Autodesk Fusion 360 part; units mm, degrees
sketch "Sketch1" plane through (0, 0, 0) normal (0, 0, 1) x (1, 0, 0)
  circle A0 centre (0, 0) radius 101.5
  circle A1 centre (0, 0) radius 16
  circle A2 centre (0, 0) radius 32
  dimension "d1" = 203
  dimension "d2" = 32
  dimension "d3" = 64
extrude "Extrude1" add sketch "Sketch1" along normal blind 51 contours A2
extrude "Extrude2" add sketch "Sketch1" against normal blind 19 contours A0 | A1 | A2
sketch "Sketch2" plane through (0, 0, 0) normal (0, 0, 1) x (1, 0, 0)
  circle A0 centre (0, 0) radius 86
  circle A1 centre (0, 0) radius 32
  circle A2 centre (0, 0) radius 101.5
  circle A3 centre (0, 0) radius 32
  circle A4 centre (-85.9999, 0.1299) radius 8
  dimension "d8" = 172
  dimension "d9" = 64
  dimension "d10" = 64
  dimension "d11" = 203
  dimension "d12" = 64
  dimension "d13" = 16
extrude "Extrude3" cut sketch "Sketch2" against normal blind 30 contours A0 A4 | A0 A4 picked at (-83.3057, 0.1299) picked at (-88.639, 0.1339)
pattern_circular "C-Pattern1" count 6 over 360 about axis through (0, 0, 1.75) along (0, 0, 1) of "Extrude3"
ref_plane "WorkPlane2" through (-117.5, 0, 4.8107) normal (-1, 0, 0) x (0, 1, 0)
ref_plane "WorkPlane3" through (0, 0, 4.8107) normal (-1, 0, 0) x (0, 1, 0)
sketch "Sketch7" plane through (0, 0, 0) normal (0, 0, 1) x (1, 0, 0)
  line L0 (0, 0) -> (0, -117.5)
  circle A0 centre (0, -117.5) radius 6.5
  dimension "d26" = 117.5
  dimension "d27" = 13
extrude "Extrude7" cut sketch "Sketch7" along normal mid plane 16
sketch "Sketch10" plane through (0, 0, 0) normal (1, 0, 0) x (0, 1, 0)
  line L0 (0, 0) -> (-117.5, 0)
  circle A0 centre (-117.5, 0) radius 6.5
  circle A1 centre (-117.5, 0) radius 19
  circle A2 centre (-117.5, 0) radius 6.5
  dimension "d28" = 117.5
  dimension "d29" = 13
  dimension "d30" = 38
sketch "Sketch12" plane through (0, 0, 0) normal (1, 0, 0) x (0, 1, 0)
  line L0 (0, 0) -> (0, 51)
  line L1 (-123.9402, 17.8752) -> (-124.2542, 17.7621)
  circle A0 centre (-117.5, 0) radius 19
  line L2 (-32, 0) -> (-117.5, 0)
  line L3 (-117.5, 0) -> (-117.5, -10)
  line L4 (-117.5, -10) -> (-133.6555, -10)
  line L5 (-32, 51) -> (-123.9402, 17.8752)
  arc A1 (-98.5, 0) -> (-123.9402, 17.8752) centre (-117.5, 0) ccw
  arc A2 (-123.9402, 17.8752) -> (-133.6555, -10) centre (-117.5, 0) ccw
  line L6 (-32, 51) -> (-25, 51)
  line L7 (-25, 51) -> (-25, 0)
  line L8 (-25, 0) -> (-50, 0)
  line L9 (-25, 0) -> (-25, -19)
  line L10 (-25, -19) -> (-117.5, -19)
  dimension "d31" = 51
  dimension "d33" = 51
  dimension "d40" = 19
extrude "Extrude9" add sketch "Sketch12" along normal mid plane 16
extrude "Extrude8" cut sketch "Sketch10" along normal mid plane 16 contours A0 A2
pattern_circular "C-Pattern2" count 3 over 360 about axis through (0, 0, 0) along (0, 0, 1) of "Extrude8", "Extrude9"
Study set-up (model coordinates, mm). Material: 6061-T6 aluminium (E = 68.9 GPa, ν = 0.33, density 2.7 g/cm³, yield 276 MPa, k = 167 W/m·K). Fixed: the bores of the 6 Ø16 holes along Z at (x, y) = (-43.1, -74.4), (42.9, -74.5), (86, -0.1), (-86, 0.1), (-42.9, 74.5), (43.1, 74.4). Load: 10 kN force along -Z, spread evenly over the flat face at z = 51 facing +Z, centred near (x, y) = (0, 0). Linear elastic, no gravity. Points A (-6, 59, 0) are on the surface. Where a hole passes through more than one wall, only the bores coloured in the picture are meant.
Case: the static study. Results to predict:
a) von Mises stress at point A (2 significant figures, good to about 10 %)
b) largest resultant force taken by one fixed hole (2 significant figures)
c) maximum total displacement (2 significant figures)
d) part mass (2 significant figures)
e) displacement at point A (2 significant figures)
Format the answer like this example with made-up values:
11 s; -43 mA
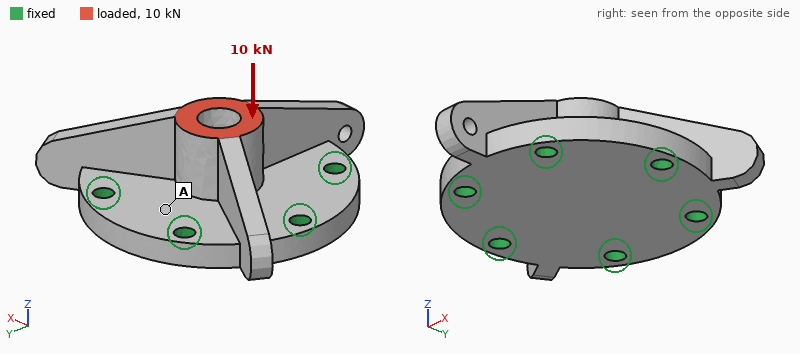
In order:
1.8 MPa; 1.8 kN; 13 µm; 2.4 kg; 4.2 µm
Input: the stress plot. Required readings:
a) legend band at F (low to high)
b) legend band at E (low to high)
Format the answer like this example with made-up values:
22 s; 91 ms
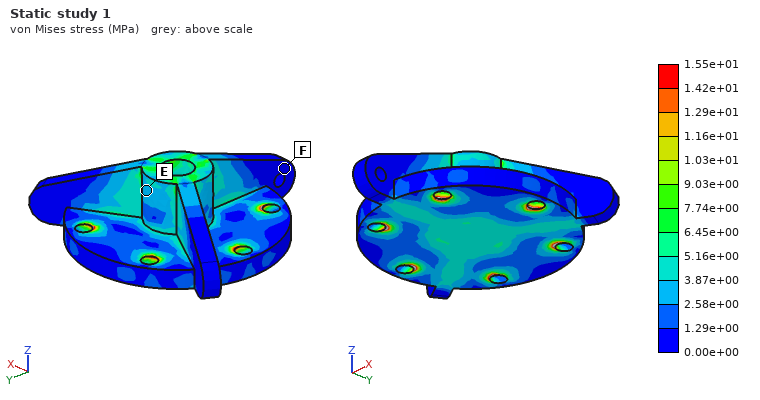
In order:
0.00e+00 to 1.29e+00 MPa; 2.58e+00 to 3.87e+00 MPa
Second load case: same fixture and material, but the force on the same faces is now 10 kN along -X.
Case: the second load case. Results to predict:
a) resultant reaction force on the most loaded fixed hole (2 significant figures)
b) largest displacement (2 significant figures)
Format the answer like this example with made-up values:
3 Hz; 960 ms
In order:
3.6 kN; 31 µm
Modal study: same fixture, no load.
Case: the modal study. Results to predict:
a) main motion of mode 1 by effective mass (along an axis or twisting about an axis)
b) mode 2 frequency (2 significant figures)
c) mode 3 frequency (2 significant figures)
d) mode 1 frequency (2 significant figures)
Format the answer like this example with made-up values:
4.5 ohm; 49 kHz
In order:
along Z; 5300 Hz; 5400 Hz; 5000 Hz
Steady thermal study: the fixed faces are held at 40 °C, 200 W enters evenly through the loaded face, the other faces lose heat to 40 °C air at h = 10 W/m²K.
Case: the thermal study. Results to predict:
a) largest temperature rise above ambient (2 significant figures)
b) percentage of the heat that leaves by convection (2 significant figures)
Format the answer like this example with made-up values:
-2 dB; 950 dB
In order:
28 K; 3.4 %
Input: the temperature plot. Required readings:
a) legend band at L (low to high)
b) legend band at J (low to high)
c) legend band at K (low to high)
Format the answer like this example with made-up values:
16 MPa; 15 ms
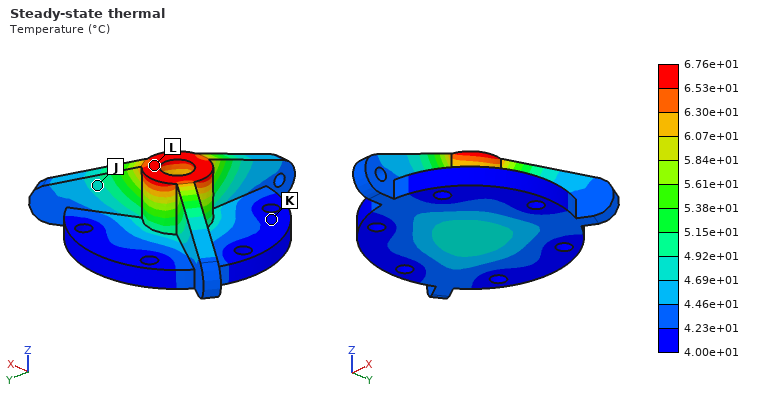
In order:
6.53e+01 to 6.76e+01 °C; 4.69e+01 to 4.92e+01 °C; 4.00e+01 to 4.23e+01 °C
